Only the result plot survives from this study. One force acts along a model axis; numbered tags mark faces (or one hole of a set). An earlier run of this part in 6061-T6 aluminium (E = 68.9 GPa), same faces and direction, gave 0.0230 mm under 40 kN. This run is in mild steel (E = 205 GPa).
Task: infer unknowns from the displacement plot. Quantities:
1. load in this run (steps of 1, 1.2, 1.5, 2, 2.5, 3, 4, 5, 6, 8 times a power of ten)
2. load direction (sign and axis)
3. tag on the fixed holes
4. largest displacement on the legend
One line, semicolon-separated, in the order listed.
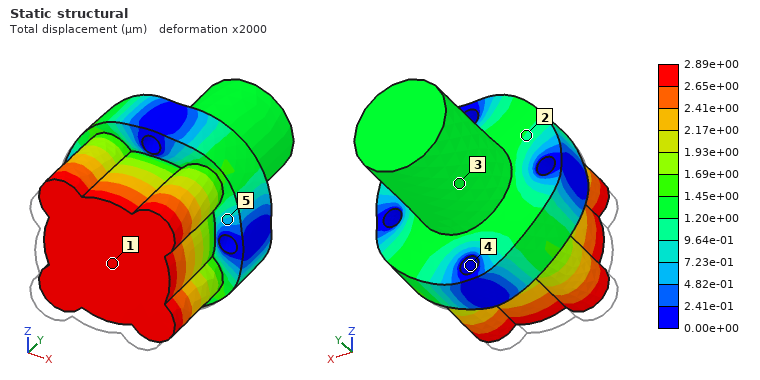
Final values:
15 kN; +Y; 4; 2.89e+00 µm
